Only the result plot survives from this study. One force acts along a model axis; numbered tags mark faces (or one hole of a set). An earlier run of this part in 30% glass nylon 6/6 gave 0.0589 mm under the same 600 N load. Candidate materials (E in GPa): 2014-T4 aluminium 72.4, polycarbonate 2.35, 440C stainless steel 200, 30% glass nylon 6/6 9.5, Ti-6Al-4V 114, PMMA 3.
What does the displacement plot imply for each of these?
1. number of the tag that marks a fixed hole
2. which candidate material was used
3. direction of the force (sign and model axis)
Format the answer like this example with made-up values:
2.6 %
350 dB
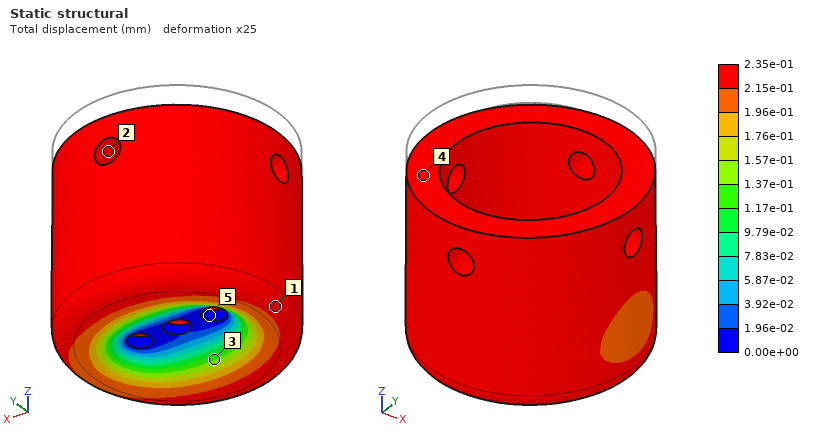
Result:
5
polycarbonate
-Z
